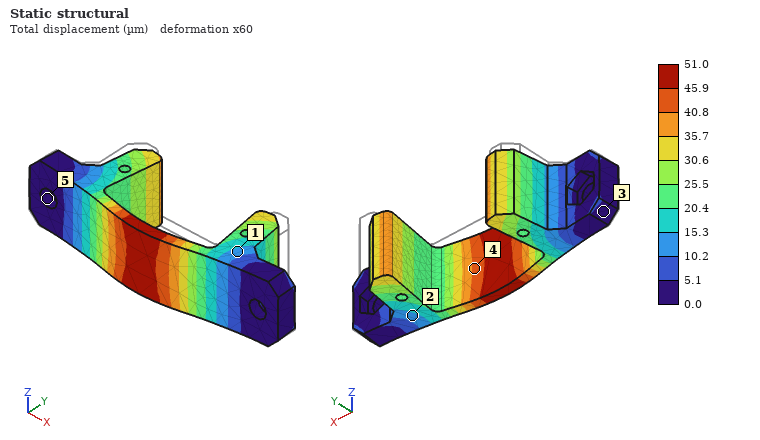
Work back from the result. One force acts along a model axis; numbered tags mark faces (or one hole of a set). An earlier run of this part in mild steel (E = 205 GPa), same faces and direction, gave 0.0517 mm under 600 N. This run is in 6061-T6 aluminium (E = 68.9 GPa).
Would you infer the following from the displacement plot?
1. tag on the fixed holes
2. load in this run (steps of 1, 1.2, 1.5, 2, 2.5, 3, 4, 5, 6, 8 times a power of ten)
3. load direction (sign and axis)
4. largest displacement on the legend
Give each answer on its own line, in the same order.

5
200 N
-Y
51.0 µm
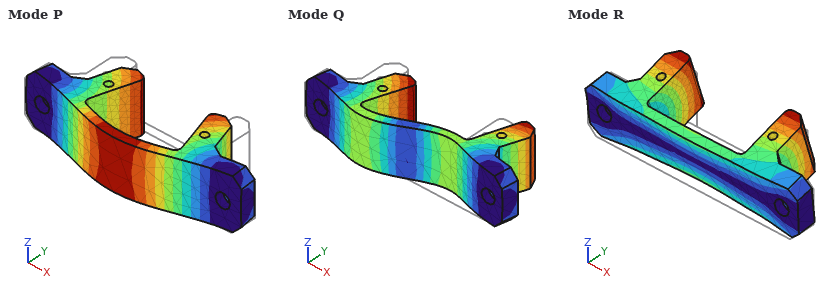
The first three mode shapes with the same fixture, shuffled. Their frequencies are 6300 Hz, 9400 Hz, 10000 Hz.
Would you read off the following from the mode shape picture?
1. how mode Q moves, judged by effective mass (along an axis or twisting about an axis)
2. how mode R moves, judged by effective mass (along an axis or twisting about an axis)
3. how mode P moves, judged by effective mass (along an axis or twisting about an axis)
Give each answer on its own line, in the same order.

along X
along Z
along Y
